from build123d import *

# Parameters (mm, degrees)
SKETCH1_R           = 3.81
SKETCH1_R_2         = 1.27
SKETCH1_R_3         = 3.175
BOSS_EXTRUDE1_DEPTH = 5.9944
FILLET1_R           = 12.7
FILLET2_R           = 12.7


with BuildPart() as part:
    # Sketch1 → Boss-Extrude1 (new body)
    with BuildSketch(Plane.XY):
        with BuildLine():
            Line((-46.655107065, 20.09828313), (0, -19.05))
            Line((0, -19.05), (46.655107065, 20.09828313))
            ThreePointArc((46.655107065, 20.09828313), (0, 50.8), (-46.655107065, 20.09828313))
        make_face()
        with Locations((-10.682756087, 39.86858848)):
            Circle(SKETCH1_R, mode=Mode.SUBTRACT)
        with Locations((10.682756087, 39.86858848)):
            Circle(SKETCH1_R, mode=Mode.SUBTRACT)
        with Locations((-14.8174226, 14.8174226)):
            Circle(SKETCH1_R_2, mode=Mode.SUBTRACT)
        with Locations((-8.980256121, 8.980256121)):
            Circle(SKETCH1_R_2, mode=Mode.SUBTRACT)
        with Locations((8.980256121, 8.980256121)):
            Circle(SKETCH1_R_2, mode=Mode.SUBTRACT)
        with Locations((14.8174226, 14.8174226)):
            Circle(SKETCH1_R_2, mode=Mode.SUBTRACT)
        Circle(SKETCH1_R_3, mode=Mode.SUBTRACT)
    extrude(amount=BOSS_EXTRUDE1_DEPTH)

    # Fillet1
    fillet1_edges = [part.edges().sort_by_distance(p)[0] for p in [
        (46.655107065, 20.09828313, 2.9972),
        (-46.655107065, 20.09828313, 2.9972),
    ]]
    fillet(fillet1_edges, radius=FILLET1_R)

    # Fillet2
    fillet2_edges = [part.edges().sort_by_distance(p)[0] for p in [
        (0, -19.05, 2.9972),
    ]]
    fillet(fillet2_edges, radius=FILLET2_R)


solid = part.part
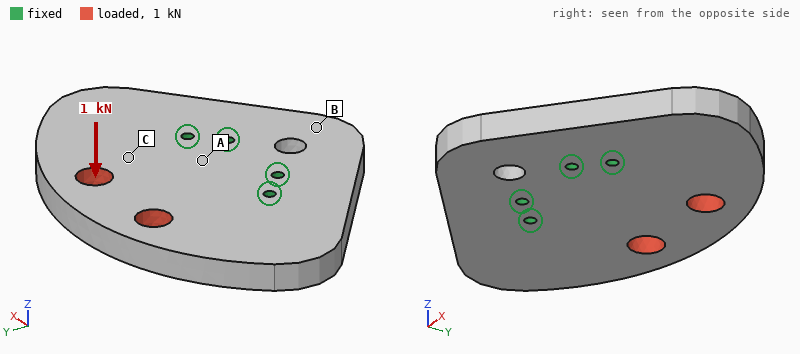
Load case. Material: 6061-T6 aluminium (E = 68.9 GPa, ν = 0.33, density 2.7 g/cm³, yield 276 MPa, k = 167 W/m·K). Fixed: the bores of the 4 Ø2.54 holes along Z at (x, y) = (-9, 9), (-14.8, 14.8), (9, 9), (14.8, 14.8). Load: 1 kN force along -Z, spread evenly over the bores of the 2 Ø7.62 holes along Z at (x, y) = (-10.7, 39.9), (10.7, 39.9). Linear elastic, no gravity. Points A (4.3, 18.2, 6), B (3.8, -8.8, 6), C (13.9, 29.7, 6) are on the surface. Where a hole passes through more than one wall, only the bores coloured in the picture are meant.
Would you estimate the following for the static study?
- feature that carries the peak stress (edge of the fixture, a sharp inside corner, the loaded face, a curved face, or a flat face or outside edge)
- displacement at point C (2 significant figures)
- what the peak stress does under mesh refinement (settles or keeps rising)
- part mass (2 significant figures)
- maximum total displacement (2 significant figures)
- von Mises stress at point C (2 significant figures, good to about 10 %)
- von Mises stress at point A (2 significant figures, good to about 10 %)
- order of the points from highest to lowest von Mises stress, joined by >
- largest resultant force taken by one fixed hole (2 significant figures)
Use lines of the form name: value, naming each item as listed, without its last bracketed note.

feature that carries the peak stress: edge of the fixture
displacement at point C: 0.047 mm
what the peak stress does under mesh refinement: keeps rising
part mass: 60 g
maximum total displacement: 0.15 mm
von Mises stress at point C: 24 MPa
von Mises stress at point A: 45 MPa
order of the points from highest to lowest von Mises stress, joined by >: A > C > B
largest resultant force taken by one fixed hole: 850 N
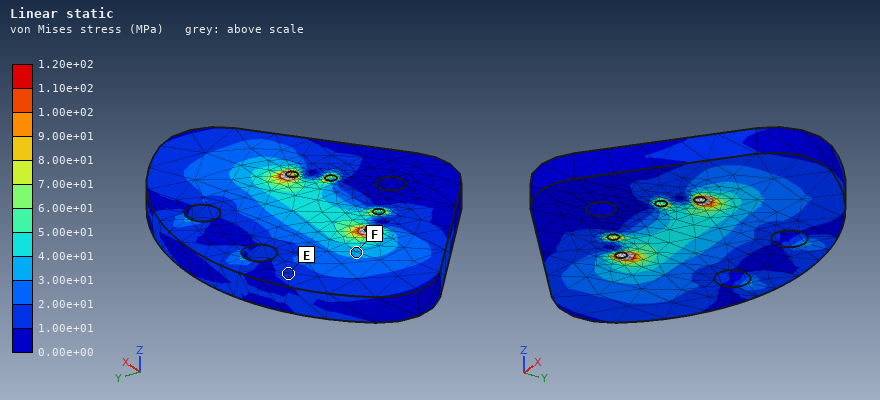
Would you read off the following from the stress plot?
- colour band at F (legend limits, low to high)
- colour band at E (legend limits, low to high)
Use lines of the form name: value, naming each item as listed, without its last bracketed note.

colour band at F: 3.00e+01 to 4.00e+01 MPa
colour band at E: 1.00e+01 to 2.00e+01 MPa
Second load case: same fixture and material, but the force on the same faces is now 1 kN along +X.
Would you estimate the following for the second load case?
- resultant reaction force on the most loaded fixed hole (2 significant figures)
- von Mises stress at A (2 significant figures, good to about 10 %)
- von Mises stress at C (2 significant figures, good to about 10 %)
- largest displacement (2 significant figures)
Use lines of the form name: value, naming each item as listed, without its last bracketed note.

resultant reaction force on the most loaded fixed hole: 860 N
von Mises stress at A: 7.2 MPa
von Mises stress at C: 5.4 MPa
largest displacement: 8.0 µm
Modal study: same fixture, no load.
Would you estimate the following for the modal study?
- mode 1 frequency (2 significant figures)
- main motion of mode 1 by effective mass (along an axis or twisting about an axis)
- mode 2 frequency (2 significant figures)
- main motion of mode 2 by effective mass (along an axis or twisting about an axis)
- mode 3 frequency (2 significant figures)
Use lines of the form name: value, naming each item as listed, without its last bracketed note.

mode 1 frequency: 3900 Hz
main motion of mode 1 by effective mass: along Z
mode 2 frequency: 5000 Hz
main motion of mode 2 by effective mass: twisting about Y
mode 3 frequency: 6300 Hz
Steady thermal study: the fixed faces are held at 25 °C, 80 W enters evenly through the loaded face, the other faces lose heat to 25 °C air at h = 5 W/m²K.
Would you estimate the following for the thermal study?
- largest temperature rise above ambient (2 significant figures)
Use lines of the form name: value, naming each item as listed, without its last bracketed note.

largest temperature rise above ambient: 47 K
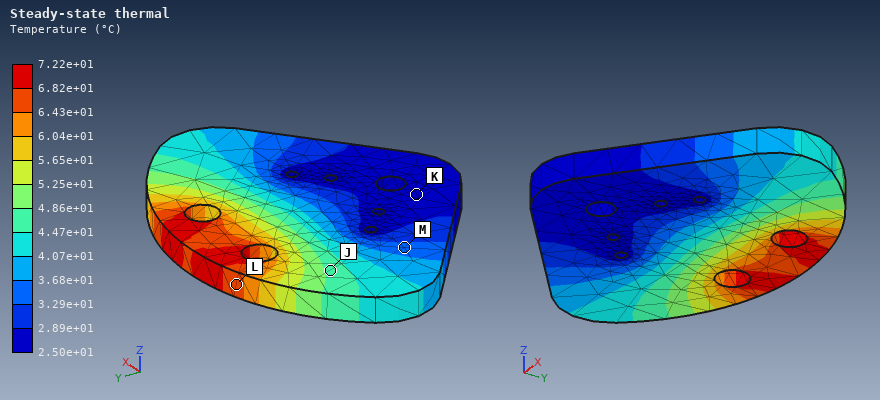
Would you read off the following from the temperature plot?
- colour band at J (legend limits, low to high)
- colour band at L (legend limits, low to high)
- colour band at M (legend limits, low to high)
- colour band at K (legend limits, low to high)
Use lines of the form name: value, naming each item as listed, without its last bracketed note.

colour band at J: 4.47e+01 to 4.86e+01 °C
colour band at L: 6.43e+01 to 6.82e+01 °C
colour band at M: 3.29e+01 to 3.68e+01 °C
colour band at K: 2.50e+01 to 2.89e+01 °C
